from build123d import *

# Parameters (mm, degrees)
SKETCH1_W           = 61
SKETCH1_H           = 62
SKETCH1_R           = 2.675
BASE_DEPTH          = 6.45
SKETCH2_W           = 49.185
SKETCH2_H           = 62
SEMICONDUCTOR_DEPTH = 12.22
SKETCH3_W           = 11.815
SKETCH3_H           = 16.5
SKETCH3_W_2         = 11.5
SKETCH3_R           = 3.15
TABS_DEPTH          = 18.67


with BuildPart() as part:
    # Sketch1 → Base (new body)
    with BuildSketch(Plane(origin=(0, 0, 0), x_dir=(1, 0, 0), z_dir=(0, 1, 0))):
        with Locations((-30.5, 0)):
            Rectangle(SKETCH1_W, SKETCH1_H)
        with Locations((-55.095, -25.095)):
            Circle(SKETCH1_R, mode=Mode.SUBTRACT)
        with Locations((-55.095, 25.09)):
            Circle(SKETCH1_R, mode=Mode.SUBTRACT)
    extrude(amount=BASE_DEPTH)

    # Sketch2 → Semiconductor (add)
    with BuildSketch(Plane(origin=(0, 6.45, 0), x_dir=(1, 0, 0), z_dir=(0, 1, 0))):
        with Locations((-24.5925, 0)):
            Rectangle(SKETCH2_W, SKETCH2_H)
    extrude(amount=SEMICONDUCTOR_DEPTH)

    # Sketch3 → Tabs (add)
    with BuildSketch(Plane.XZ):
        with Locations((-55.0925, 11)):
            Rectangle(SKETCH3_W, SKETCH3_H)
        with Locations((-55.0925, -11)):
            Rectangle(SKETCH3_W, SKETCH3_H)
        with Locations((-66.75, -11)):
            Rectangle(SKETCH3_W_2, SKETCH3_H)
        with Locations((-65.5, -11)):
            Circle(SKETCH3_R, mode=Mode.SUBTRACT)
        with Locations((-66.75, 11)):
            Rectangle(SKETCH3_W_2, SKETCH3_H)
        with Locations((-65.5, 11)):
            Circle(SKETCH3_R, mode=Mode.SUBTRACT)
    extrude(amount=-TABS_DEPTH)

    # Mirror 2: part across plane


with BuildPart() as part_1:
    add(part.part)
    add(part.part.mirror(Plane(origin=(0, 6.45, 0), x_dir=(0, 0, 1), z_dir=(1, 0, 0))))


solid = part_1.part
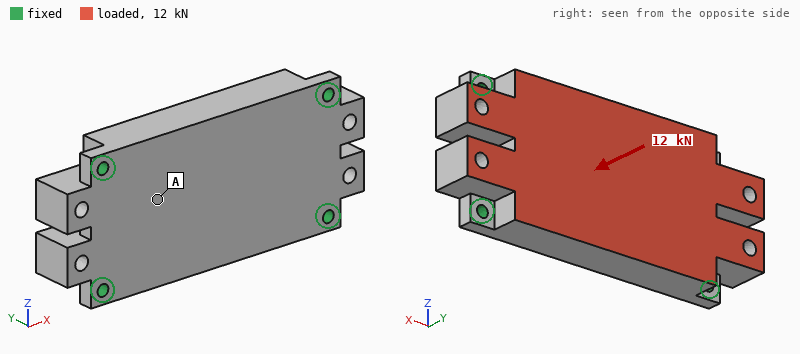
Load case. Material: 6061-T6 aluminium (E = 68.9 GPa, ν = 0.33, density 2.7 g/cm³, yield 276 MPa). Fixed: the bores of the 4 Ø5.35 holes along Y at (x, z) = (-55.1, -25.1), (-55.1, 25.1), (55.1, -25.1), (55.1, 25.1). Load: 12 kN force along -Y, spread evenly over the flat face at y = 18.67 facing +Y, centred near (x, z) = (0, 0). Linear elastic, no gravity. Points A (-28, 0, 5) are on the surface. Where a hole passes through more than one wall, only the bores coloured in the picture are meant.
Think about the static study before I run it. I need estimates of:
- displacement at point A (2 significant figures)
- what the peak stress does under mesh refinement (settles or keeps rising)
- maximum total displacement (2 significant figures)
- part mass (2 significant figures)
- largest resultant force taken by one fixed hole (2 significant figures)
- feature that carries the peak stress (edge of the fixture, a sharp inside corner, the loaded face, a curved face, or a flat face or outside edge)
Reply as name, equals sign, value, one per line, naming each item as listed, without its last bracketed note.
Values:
displacement at point A = 37 µm
what the peak stress does under mesh refinement = keeps rising
maximum total displacement = 53 µm
part mass = 390 g
largest resultant force taken by one fixed hole = 4.0 kN
feature that carries the peak stress = edge of the fixture
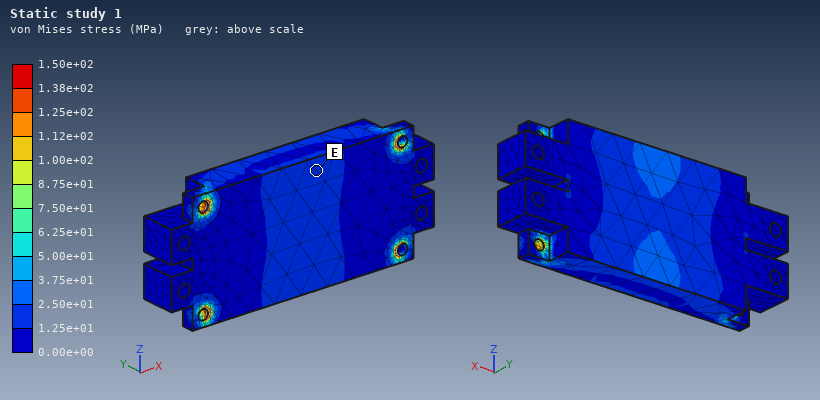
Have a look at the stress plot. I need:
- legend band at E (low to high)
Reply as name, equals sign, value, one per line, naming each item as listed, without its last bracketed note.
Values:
legend band at E = 1.25e+01 to 2.50e+01 MPa
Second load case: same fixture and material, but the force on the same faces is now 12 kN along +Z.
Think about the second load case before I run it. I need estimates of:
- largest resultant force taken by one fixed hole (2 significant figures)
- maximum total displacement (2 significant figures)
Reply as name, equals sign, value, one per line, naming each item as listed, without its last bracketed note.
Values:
largest resultant force taken by one fixed hole = 4.0 kN
maximum total displacement = 26 µm
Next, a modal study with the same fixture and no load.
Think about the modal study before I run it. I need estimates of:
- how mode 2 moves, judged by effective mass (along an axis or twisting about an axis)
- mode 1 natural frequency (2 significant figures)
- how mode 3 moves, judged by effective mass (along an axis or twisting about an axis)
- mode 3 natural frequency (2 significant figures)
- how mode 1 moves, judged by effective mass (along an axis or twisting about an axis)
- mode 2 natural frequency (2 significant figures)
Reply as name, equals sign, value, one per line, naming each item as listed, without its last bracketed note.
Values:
how mode 2 moves, judged by effective mass = twisting about X
mode 1 natural frequency = 4300 Hz
how mode 3 moves, judged by effective mass = along Z
mode 3 natural frequency = 8700 Hz
how mode 1 moves, judged by effective mass = along Y
mode 2 natural frequency = 7300 Hz
